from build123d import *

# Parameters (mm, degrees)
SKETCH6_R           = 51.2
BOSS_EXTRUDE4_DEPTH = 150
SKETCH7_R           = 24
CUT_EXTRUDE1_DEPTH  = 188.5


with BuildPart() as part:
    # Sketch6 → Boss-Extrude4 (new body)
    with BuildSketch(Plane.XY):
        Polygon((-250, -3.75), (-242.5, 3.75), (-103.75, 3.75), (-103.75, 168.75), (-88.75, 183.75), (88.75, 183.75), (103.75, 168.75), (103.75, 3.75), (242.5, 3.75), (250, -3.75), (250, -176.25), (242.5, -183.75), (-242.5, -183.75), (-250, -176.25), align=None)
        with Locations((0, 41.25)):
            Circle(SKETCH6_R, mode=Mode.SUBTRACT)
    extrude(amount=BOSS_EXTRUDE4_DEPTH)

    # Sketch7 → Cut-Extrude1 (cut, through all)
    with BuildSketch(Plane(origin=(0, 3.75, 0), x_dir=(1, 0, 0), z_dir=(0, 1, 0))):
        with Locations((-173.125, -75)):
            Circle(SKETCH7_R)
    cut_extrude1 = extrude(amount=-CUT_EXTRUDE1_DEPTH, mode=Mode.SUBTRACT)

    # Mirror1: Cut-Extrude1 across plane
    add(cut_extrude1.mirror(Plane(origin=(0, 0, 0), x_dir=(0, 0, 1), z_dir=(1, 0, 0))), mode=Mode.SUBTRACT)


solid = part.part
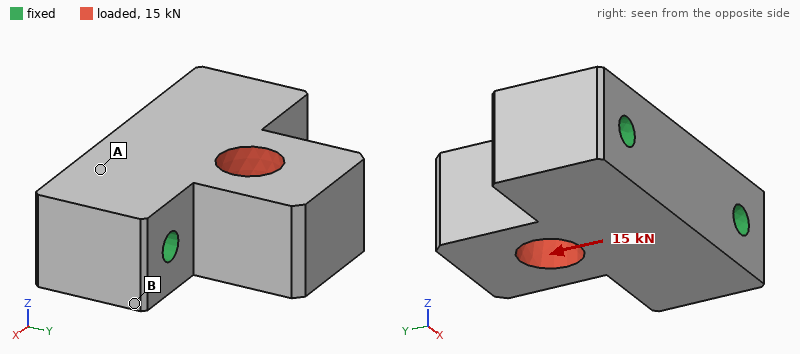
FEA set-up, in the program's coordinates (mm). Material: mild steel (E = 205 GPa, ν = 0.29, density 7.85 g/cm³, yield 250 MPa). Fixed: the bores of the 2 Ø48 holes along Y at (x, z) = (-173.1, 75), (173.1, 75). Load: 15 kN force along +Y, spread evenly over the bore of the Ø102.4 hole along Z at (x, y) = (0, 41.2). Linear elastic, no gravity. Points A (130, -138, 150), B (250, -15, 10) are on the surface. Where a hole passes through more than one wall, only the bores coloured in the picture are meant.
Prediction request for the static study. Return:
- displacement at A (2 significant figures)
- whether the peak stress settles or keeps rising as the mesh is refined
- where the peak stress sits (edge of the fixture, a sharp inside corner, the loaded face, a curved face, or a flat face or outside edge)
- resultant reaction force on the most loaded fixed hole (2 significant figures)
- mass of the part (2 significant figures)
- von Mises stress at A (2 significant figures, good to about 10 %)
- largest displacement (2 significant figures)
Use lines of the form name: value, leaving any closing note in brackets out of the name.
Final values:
displacement at A: 0.17 µm
whether the peak stress settles or keeps rising as the mesh is refined: keeps rising
where the peak stress sits: edge of the fixture
resultant reaction force on the most loaded fixed hole: 7.7 kN
mass of the part: 140 kg
von Mises stress at A: 0.33 MPa
largest displacement: 0.80 µm
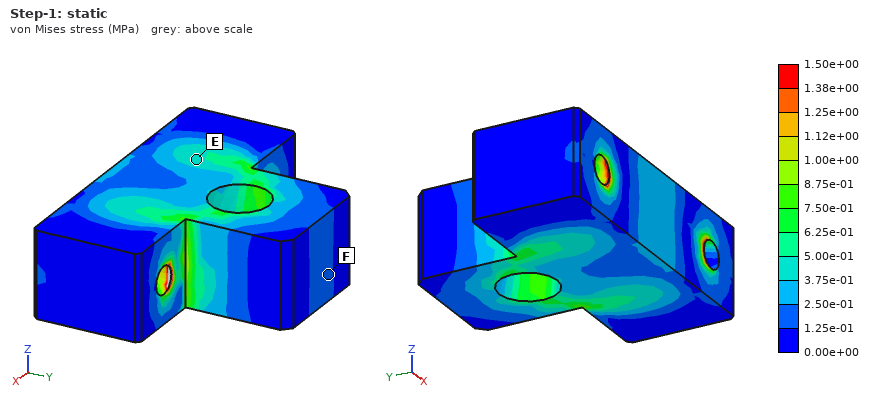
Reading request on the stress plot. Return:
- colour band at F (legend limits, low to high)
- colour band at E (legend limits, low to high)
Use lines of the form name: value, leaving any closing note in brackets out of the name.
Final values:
colour band at F: 1.25e-01 to 2.50e-01 MPa
colour band at E: 3.75e-01 to 5.00e-01 MPa
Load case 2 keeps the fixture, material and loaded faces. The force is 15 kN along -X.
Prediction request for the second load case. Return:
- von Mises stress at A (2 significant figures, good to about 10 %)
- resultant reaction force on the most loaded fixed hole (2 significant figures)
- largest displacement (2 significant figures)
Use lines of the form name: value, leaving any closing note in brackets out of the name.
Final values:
von Mises stress at A: 0.15 MPa
resultant reaction force on the most loaded fixed hole: 9.0 kN
largest displacement: 2.0 µm
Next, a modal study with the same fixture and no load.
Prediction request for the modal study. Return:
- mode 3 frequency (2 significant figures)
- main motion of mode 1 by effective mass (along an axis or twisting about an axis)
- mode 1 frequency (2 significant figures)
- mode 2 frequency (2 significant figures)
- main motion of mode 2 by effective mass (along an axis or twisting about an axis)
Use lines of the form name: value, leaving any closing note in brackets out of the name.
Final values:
mode 3 frequency: 2500 Hz
main motion of mode 1 by effective mass: along Z
mode 1 frequency: 1200 Hz
mode 2 frequency: 1800 Hz
main motion of mode 2 by effective mass: along X
